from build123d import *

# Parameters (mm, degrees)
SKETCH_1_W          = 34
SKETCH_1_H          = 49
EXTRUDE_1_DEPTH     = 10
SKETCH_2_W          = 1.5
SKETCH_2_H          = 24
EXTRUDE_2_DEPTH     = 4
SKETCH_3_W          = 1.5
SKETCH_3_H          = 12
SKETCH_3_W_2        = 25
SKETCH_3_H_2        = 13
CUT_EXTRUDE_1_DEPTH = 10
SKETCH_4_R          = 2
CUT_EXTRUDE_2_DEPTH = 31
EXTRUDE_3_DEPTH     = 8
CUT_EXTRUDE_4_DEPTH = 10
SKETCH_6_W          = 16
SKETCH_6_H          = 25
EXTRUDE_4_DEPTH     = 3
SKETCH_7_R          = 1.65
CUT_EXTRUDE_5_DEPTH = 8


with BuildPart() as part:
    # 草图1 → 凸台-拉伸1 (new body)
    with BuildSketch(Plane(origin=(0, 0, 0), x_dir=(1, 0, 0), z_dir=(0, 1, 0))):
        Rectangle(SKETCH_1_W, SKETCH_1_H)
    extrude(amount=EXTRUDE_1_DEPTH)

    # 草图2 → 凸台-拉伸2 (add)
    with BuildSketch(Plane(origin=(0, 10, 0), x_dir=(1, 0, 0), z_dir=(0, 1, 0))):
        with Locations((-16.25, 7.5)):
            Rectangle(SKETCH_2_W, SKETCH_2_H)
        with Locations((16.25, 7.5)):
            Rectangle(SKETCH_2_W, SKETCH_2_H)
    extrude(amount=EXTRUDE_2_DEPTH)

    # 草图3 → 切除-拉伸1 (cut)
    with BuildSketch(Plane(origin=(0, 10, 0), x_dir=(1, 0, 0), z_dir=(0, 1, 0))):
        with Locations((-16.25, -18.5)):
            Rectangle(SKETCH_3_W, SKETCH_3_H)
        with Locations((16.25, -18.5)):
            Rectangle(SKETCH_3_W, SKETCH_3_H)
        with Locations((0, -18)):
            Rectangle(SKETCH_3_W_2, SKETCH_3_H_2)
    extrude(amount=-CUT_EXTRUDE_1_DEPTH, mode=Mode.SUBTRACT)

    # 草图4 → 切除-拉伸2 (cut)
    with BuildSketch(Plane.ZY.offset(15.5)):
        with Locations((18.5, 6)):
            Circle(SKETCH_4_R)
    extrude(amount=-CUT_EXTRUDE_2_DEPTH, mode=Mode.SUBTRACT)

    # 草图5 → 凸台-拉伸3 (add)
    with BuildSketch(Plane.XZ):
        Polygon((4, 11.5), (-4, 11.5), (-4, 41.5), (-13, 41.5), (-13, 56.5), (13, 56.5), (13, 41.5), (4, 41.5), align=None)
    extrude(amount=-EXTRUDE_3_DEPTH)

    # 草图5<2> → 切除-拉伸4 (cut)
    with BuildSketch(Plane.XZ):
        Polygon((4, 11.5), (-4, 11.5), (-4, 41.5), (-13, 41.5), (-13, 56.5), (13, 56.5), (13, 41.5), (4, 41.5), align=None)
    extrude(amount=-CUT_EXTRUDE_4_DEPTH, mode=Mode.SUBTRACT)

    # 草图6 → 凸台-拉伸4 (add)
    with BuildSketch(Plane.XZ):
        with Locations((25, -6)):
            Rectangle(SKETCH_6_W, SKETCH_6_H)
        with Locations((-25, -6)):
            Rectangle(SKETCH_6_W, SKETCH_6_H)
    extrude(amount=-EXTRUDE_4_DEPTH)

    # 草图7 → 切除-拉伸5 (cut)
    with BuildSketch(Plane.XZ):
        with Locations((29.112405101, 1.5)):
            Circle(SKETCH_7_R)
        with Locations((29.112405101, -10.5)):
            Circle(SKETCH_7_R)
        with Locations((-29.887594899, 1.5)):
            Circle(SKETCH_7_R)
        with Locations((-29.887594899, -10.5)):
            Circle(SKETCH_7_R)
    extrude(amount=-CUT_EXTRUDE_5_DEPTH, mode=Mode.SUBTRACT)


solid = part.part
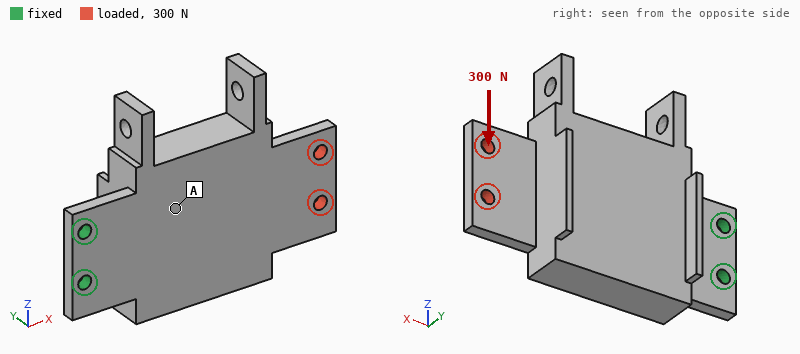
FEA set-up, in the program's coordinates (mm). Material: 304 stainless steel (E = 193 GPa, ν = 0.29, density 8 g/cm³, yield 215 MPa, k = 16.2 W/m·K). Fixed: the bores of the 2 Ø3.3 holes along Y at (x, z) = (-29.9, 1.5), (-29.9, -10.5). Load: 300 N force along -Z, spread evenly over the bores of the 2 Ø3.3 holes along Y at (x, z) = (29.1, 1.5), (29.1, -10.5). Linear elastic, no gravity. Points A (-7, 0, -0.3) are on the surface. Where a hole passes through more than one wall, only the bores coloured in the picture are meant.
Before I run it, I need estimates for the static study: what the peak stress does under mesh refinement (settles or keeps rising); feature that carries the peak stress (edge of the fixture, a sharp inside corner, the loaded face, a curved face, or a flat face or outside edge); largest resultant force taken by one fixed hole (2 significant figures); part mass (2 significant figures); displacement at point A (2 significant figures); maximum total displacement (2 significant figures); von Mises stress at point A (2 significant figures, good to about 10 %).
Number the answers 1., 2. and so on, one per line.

1. keeps rising
2. edge of the fixture
3. 1.2 kN
4. 120 g
5. 9.9 µm
6. 33 µm
7. 12 MPa
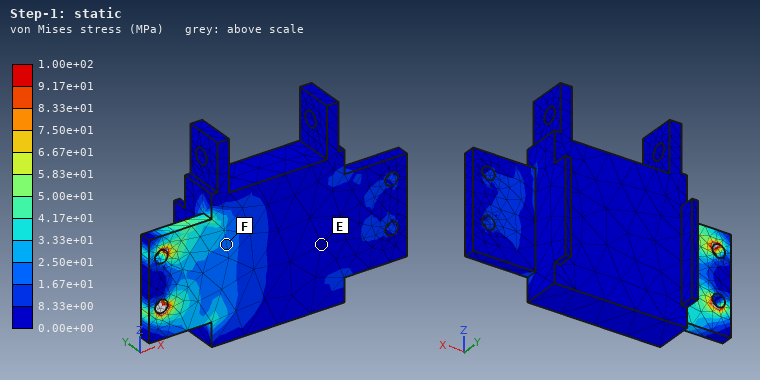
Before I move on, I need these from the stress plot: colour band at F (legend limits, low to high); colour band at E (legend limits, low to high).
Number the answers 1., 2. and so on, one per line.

1. 1.67e+01 to 2.50e+01 MPa
2. 0.00e+00 to 8.33e+00 MPa
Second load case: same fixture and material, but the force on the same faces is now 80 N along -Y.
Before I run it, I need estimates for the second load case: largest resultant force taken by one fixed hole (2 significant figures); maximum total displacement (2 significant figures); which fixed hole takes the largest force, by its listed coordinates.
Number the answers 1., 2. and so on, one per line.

1. 47 N
2. 0.30 mm
3. (-29.9, -10.5)
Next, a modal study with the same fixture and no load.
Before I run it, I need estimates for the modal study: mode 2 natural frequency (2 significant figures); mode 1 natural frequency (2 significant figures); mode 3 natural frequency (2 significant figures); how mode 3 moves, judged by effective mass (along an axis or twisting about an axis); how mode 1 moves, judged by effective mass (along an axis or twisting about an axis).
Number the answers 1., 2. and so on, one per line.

1. 2000 Hz
2. 480 Hz
3. 2700 Hz
4. along Z
5. along Y
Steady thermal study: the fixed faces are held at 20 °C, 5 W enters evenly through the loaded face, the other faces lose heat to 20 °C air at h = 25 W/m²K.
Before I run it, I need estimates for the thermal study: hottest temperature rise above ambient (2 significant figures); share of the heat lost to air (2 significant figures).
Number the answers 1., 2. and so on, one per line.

1. 86 K
2. 77 %
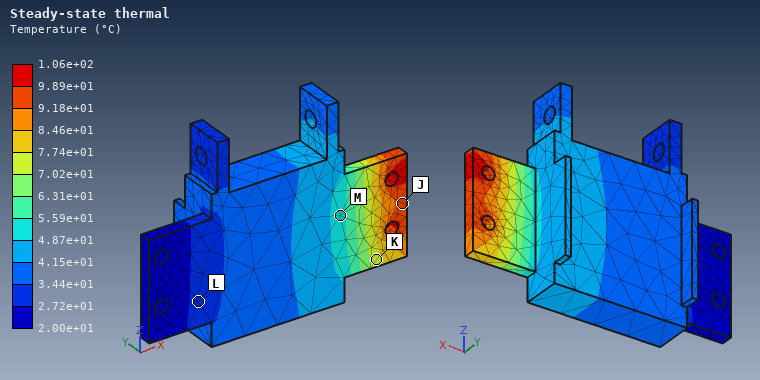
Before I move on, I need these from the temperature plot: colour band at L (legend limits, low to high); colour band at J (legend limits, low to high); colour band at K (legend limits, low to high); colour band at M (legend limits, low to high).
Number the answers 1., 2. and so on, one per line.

1. 2.72e+01 to 3.44e+01 °C
2. 9.18e+01 to 9.89e+01 °C
3. 7.02e+01 to 7.74e+01 °C
4. 4.87e+01 to 5.59e+01 °C
